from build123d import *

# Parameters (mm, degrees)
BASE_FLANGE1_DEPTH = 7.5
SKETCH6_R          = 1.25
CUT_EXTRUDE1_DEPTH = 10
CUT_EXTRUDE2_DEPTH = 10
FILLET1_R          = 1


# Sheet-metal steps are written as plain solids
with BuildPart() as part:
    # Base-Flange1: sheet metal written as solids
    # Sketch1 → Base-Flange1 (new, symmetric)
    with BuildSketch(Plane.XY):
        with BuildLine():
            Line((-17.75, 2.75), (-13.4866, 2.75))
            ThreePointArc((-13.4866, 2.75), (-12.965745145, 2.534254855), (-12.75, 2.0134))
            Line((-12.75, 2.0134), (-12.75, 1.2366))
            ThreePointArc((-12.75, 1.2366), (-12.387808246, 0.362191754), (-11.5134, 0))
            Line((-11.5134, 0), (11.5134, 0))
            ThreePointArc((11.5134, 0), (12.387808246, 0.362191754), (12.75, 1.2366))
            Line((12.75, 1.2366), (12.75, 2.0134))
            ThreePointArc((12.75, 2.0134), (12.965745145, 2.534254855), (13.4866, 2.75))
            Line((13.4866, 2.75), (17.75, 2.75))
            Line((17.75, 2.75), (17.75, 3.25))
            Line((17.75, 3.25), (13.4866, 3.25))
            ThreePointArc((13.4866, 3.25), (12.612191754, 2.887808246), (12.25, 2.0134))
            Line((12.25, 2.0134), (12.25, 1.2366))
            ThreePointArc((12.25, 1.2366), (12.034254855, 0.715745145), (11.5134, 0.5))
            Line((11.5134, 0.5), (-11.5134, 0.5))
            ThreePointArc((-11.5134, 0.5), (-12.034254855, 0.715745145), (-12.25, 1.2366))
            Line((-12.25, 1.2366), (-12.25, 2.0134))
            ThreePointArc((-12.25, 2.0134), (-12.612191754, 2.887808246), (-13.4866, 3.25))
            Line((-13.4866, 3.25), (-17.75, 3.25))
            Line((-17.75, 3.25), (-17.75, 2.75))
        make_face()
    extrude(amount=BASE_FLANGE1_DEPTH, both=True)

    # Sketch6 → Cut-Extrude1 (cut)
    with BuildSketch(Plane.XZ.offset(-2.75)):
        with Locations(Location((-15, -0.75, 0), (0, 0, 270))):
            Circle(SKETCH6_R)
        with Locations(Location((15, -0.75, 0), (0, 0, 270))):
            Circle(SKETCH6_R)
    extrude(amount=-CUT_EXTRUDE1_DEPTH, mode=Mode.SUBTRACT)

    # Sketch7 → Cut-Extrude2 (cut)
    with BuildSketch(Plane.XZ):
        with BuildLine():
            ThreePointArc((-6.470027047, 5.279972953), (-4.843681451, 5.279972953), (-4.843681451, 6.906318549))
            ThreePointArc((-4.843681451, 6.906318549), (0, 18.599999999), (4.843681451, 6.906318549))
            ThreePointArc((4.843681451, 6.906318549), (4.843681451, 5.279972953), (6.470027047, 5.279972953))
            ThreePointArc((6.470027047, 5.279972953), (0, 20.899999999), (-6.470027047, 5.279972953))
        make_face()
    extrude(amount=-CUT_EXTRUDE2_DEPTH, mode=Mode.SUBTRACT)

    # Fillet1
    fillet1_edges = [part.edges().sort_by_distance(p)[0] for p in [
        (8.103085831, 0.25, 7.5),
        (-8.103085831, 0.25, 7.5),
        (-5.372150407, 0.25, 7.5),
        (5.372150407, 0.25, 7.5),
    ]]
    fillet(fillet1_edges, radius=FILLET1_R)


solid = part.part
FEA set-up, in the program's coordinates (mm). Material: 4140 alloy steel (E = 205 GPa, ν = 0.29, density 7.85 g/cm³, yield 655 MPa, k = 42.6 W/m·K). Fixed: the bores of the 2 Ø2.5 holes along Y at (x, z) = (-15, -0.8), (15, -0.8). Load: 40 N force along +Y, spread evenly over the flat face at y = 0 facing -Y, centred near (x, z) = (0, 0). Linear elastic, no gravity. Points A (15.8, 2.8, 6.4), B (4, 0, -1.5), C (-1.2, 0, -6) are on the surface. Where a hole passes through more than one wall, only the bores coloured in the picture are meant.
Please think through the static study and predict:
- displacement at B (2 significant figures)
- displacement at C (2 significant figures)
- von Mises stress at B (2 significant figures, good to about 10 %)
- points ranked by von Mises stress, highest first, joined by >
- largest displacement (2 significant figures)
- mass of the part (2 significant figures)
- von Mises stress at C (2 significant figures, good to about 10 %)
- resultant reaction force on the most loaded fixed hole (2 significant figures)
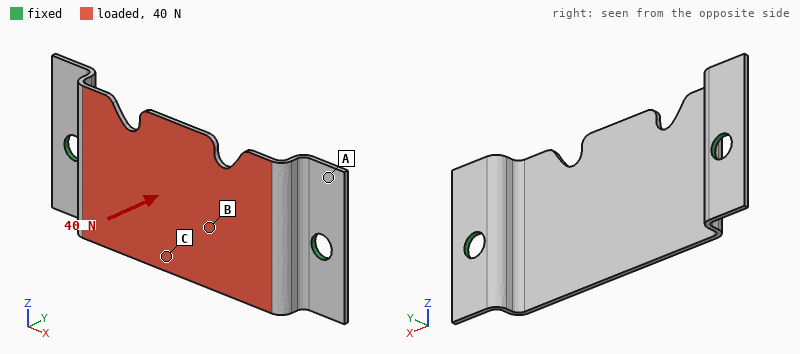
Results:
48 µm
59 µm
57 MPa
C > B > A
69 µm
2.2 g
78 MPa
47 N
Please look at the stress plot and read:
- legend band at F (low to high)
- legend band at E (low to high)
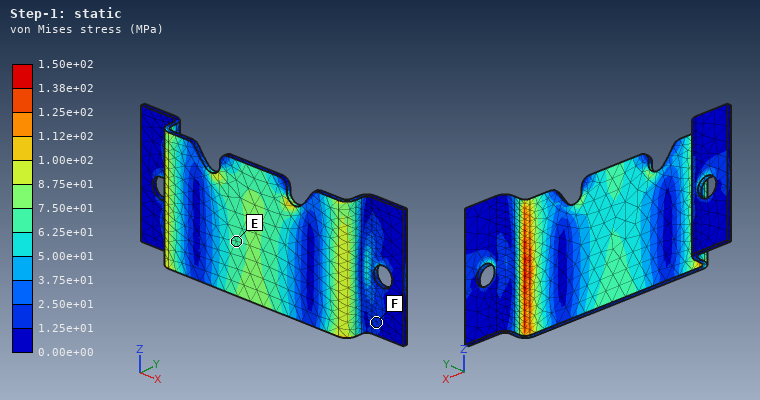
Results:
1.25e+01 to 2.50e+01 MPa
6.25e+01 to 7.50e+01 MPa
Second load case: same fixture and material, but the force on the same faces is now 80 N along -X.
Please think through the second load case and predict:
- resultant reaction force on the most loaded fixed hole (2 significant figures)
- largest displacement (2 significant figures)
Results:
40 N
24 µm
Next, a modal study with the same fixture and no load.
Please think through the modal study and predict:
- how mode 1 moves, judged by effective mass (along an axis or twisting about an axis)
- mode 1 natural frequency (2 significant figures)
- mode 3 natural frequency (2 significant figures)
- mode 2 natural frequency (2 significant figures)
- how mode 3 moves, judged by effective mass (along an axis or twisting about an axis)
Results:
along Y
4100 Hz
6800 Hz
5100 Hz
along X
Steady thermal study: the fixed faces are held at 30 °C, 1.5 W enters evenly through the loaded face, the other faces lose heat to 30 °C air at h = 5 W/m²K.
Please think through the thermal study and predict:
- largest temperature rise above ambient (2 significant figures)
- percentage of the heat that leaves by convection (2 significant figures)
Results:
31 K
4.3 %
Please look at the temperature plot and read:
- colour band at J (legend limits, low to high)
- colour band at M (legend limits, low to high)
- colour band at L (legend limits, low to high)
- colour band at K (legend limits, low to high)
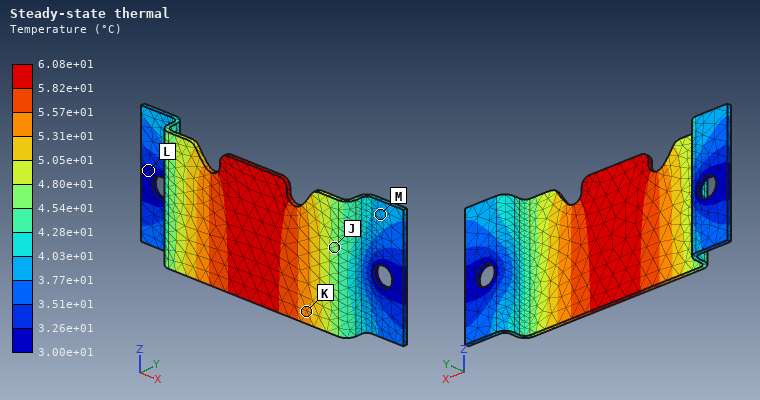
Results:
4.54e+01 to 4.80e+01 °C
3.77e+01 to 4.03e+01 °C
3.00e+01 to 3.26e+01 °C
5.31e+01 to 5.57e+01 °C
